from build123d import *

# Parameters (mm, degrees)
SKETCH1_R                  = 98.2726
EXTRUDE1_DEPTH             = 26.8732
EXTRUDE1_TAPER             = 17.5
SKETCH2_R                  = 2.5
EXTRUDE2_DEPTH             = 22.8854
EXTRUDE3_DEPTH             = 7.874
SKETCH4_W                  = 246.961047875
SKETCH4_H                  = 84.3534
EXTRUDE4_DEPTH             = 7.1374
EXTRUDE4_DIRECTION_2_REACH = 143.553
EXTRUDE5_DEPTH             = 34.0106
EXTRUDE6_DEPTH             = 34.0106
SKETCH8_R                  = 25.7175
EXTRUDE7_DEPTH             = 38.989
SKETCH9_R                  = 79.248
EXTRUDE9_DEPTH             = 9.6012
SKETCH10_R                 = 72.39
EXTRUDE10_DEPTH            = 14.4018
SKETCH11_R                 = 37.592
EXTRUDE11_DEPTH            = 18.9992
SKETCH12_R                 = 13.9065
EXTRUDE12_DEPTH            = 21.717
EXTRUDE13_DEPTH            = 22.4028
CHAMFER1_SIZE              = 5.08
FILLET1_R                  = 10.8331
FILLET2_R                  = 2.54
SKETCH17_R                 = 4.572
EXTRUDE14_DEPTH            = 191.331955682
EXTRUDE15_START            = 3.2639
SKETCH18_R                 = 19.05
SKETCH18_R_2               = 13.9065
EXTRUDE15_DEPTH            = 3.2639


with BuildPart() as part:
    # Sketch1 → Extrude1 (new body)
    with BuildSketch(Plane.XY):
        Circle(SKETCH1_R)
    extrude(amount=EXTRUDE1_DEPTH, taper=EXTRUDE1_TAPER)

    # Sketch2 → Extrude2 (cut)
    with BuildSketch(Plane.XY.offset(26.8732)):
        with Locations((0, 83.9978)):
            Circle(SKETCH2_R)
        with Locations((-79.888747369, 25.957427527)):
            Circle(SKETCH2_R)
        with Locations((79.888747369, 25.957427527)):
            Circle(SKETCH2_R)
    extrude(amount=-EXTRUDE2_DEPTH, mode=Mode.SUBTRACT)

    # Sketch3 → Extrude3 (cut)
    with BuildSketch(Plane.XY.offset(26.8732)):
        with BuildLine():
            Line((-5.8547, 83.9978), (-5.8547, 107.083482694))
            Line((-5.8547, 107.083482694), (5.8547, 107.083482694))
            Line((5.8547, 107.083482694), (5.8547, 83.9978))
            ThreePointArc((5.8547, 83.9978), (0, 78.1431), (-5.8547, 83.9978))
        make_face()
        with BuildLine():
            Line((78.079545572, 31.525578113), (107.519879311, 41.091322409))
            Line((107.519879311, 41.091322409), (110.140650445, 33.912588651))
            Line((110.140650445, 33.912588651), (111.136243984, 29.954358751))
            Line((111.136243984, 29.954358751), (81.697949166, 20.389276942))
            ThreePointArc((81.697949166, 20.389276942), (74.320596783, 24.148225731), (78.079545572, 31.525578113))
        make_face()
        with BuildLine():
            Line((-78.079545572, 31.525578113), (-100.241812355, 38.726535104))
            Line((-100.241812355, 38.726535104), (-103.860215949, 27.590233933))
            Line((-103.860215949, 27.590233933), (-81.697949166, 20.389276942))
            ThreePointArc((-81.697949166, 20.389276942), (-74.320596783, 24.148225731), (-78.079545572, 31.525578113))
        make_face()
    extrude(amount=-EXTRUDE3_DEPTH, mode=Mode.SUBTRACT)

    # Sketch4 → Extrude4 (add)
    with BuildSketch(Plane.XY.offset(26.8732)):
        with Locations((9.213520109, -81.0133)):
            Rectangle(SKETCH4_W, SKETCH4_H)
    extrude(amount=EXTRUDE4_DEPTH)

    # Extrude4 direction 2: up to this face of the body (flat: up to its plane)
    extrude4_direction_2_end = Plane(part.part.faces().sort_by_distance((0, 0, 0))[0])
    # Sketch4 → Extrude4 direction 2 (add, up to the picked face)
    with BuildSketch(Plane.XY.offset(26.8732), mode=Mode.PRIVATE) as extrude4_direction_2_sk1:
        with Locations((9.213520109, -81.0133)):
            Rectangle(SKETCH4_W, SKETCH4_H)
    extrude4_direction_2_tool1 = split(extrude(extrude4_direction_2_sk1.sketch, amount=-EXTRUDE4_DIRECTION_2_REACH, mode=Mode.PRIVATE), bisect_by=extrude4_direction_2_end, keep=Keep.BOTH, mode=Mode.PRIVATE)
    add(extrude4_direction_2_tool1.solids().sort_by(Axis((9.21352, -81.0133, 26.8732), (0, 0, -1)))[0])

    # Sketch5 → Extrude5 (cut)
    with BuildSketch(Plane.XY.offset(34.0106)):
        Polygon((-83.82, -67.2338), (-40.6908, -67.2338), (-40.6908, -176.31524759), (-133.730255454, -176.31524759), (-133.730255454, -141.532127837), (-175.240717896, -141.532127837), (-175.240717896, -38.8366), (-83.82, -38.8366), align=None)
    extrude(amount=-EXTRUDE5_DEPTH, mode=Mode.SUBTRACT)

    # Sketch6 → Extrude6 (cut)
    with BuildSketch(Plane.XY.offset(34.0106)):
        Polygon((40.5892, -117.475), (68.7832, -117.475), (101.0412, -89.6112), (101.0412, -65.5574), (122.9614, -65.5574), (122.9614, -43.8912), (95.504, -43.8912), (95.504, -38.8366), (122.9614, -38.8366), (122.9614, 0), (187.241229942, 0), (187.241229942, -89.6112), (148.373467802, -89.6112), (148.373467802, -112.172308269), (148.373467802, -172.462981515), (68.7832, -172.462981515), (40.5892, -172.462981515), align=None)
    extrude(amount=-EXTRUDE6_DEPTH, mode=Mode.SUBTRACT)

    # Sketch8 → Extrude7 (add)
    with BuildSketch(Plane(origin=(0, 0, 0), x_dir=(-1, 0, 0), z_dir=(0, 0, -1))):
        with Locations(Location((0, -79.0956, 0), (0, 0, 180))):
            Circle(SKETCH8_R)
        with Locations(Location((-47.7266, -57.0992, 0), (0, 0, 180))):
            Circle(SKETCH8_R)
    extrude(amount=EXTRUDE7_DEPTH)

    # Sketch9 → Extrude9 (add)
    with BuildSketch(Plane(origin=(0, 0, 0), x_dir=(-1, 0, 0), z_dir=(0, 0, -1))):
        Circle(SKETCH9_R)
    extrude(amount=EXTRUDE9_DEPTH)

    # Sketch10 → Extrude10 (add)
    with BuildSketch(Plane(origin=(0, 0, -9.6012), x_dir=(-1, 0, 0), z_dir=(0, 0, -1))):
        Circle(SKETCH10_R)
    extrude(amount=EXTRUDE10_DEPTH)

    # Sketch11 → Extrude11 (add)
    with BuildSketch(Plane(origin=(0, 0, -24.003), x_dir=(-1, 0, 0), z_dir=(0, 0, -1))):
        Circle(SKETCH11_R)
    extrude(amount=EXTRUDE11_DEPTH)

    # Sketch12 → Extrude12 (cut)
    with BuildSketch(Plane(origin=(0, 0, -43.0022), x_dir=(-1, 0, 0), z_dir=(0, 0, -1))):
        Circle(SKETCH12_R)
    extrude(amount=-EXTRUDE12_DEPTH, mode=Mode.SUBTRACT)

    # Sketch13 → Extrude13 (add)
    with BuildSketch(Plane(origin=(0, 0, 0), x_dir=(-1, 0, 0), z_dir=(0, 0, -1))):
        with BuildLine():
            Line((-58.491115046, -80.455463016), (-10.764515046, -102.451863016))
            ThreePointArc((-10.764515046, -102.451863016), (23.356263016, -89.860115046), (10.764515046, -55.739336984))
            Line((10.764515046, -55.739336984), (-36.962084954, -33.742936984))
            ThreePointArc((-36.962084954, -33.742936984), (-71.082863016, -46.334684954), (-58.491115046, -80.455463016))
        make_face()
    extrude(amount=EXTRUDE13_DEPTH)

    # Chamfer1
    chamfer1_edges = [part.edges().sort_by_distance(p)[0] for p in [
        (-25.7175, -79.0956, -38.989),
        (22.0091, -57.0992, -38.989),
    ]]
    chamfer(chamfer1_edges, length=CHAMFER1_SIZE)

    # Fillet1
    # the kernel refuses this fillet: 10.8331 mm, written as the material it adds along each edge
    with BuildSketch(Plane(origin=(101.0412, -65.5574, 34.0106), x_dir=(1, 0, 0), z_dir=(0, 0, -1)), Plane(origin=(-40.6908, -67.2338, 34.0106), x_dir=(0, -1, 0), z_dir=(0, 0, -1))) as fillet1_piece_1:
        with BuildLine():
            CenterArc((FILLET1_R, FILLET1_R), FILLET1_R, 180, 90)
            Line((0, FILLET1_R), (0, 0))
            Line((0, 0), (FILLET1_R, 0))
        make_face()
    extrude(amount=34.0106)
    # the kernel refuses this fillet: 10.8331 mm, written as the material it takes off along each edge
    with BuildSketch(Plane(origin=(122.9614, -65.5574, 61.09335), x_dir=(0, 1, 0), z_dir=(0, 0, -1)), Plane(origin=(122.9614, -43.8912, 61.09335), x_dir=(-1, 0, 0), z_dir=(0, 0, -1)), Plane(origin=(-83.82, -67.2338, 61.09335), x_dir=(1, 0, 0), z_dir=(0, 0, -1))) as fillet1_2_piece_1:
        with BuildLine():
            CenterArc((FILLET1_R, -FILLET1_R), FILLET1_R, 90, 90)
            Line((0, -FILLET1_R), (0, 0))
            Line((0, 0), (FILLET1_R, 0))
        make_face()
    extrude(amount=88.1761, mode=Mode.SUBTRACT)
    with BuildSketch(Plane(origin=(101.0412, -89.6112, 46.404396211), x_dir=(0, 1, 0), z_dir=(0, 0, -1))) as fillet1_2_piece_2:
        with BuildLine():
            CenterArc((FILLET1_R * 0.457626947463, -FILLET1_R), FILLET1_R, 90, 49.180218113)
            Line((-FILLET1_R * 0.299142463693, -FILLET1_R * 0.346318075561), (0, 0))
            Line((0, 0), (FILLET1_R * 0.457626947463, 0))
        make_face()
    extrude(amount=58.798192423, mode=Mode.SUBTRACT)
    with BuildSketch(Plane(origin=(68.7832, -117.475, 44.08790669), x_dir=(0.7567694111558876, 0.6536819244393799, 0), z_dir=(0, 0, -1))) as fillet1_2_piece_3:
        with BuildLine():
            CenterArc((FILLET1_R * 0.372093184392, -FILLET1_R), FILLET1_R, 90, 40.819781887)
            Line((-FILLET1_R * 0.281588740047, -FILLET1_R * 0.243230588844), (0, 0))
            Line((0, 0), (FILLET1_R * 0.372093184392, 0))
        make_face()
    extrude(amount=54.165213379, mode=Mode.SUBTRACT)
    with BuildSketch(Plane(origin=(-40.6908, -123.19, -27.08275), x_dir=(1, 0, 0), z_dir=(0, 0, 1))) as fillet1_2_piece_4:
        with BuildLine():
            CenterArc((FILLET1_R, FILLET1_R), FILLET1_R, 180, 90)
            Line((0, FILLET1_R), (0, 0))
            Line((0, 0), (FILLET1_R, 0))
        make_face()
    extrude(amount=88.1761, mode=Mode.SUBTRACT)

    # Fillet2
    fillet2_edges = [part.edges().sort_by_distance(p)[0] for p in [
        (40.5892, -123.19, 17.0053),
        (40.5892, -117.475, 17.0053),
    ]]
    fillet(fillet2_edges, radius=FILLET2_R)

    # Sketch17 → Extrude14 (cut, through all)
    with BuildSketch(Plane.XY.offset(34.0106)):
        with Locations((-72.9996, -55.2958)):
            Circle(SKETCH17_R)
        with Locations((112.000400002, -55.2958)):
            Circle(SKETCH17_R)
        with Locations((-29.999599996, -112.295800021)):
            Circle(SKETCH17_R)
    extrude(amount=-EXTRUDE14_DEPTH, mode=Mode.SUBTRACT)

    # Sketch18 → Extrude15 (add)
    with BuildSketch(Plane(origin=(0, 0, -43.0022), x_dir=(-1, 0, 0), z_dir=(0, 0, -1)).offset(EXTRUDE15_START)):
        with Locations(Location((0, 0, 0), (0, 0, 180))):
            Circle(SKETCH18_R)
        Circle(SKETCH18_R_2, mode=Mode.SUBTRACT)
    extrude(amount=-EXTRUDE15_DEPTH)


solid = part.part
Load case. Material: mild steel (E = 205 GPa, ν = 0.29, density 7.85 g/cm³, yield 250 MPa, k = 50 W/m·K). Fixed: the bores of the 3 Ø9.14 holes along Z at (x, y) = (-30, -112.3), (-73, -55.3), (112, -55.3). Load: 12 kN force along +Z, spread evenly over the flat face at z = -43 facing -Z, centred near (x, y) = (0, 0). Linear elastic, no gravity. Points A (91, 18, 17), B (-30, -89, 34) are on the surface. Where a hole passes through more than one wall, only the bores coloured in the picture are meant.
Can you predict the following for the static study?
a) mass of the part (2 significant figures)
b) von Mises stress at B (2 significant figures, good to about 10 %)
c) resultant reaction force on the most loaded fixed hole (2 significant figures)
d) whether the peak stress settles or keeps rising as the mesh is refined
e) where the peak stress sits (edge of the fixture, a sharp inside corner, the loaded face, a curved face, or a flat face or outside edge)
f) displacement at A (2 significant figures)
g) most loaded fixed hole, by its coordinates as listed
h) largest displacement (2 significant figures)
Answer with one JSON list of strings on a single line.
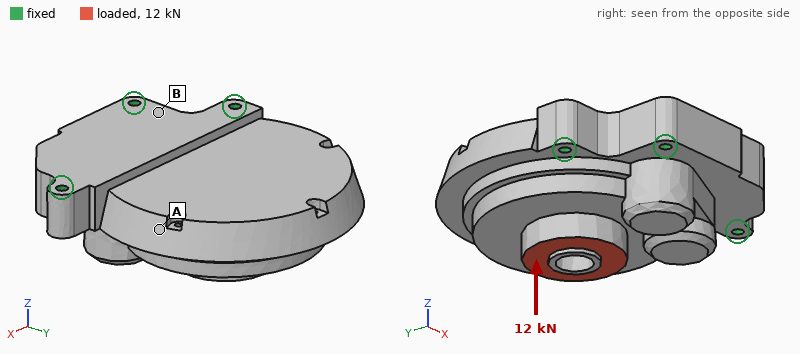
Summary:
["13 kg", "14 MPa", "11 kN", "keeps rising", "edge of the fixture", "26 µm", "(-73, -55.3)", "47 µm"]
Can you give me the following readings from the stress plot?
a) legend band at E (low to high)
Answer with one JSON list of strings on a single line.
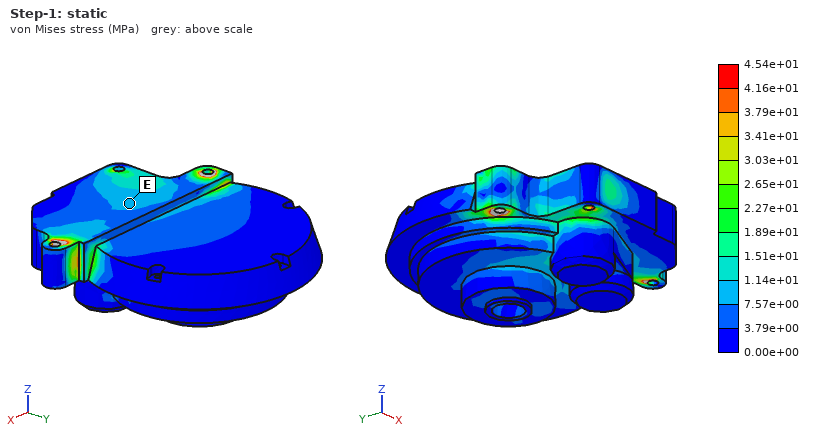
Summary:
["7.57e+00 to 1.14e+01 MPa"]
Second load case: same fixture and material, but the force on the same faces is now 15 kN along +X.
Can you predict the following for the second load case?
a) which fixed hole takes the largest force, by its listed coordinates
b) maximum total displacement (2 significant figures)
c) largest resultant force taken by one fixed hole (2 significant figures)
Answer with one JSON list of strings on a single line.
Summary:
["(-73, -55.3)", "12 µm", "11 kN"]
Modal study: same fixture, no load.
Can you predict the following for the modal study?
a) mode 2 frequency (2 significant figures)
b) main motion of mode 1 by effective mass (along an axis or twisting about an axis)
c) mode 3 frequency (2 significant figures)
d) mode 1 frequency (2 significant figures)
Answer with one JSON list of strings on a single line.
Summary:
["2700 Hz", "along Z", "3300 Hz", "1000 Hz"]
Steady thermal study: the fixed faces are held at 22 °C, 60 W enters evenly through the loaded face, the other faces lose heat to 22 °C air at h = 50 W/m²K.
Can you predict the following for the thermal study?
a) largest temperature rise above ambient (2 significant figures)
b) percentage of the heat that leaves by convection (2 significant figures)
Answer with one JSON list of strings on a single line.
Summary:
["18 K", "56 %"]
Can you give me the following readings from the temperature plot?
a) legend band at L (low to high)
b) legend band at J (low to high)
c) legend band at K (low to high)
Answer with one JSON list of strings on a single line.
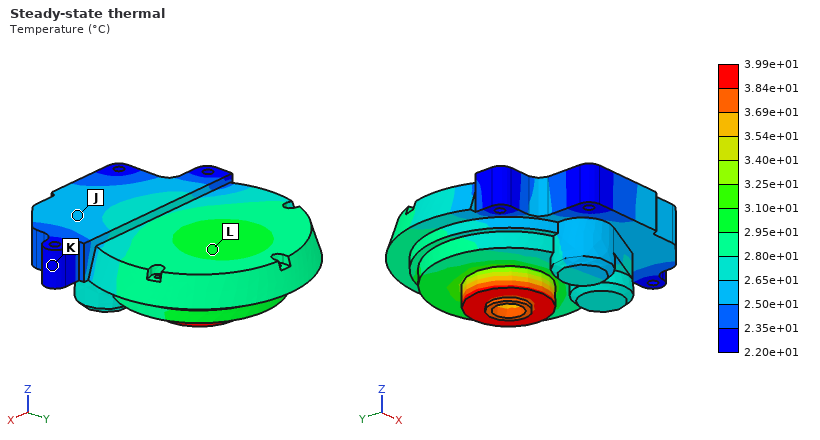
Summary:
["2.95e+01 to 3.10e+01 °C", "2.50e+01 to 2.65e+01 °C", "2.20e+01 to 2.35e+01 °C"]
